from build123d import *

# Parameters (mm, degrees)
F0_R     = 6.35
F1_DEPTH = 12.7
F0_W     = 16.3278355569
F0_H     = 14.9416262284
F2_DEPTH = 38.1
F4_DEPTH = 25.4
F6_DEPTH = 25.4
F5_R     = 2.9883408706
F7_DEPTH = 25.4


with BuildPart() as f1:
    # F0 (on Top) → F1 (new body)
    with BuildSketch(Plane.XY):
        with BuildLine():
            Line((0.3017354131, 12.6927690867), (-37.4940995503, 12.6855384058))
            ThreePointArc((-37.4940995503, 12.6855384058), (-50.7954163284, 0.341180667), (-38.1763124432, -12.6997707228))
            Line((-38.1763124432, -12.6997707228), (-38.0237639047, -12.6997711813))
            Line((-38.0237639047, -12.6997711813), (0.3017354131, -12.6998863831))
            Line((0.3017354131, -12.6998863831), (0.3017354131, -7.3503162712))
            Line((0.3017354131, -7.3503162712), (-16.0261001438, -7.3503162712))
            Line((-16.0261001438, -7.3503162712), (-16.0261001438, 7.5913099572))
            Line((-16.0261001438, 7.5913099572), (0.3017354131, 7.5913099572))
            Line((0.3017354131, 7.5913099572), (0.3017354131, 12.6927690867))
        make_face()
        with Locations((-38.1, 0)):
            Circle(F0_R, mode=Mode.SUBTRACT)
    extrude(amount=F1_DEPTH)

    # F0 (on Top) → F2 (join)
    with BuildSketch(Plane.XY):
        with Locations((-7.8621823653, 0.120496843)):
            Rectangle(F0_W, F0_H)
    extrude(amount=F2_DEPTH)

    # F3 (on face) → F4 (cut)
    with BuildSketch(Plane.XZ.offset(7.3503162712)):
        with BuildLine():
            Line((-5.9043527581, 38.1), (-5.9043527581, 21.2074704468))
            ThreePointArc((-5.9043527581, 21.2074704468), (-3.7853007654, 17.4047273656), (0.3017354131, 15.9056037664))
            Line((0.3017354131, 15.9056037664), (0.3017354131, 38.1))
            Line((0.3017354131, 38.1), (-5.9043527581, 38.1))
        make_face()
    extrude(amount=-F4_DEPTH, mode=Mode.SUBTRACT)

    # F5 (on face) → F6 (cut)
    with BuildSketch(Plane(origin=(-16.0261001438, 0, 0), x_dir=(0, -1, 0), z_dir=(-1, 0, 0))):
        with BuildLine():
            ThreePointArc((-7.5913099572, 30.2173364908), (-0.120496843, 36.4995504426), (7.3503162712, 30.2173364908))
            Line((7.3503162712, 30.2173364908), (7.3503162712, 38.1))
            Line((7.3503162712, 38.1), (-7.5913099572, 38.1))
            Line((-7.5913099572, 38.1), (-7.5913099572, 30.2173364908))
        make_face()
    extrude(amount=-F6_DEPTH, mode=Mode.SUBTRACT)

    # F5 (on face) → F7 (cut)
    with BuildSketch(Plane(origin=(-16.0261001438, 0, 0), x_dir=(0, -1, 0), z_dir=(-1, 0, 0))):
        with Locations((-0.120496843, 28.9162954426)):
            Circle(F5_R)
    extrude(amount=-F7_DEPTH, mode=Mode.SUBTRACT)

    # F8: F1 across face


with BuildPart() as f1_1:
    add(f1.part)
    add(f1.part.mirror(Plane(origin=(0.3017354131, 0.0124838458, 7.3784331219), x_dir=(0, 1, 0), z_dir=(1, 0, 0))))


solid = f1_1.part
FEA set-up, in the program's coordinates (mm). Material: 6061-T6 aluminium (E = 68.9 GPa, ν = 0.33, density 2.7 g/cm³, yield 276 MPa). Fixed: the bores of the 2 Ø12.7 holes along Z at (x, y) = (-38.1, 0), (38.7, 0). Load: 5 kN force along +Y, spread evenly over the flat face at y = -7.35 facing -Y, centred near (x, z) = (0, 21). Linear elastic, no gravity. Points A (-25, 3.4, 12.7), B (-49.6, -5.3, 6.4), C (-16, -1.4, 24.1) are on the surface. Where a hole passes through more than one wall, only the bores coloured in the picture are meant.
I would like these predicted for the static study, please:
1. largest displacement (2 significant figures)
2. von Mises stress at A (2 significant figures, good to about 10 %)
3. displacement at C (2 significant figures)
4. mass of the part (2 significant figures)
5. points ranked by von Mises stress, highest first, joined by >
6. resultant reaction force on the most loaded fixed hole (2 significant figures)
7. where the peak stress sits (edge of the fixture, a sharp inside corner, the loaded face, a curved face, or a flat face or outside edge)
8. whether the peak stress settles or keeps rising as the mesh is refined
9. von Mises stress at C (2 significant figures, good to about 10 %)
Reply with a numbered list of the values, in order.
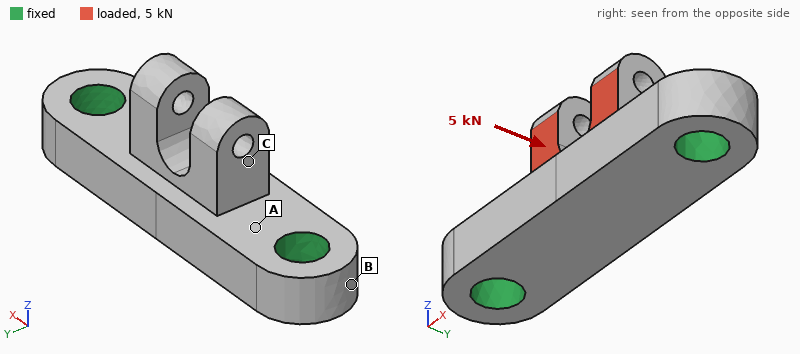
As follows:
1. 0.10 mm
2. 64 MPa
3. 0.062 mm
4. 94 g
5. A > C > B
6. 2.5 kN
7. edge of the fixture
8. keeps rising
9. 16 MPa
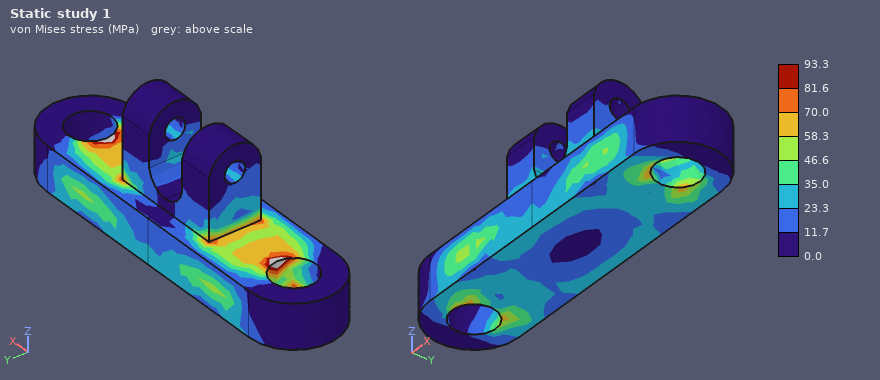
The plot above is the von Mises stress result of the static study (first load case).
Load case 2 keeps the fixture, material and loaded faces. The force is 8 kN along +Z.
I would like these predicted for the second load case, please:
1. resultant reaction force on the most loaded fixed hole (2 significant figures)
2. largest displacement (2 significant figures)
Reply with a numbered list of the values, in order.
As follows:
1. 4.1 kN
2. 95 µm
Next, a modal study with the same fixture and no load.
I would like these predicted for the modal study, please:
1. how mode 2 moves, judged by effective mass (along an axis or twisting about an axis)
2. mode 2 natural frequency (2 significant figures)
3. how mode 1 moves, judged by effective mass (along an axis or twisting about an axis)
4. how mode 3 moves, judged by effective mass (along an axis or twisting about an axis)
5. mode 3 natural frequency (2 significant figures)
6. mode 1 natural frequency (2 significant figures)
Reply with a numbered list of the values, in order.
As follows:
1. along Z
2. 10 kHz
3. along Y
4. along X
5. 14 kHz
6. 8300 Hz
